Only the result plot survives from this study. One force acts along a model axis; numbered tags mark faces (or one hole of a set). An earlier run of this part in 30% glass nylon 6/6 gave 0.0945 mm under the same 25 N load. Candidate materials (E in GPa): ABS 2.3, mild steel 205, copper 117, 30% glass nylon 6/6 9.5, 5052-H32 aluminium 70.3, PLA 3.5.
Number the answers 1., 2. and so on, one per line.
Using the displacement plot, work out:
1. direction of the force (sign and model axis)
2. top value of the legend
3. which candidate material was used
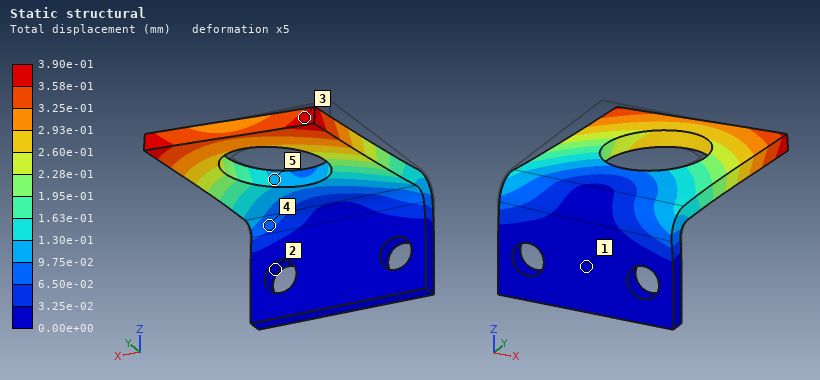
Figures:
1. +X
2. 3.90e-01 mm
3. ABS
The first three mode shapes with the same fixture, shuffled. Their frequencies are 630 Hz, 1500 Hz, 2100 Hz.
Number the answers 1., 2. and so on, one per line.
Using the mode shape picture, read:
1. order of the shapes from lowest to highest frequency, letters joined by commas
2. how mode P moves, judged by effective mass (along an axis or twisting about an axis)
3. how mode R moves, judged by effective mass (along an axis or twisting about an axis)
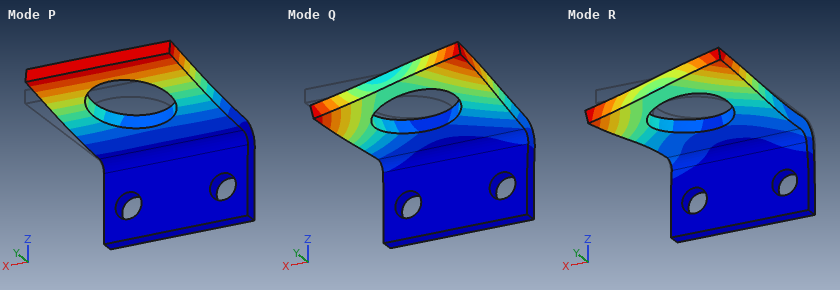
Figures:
1. P, Q, R
2. along Z
3. along X
